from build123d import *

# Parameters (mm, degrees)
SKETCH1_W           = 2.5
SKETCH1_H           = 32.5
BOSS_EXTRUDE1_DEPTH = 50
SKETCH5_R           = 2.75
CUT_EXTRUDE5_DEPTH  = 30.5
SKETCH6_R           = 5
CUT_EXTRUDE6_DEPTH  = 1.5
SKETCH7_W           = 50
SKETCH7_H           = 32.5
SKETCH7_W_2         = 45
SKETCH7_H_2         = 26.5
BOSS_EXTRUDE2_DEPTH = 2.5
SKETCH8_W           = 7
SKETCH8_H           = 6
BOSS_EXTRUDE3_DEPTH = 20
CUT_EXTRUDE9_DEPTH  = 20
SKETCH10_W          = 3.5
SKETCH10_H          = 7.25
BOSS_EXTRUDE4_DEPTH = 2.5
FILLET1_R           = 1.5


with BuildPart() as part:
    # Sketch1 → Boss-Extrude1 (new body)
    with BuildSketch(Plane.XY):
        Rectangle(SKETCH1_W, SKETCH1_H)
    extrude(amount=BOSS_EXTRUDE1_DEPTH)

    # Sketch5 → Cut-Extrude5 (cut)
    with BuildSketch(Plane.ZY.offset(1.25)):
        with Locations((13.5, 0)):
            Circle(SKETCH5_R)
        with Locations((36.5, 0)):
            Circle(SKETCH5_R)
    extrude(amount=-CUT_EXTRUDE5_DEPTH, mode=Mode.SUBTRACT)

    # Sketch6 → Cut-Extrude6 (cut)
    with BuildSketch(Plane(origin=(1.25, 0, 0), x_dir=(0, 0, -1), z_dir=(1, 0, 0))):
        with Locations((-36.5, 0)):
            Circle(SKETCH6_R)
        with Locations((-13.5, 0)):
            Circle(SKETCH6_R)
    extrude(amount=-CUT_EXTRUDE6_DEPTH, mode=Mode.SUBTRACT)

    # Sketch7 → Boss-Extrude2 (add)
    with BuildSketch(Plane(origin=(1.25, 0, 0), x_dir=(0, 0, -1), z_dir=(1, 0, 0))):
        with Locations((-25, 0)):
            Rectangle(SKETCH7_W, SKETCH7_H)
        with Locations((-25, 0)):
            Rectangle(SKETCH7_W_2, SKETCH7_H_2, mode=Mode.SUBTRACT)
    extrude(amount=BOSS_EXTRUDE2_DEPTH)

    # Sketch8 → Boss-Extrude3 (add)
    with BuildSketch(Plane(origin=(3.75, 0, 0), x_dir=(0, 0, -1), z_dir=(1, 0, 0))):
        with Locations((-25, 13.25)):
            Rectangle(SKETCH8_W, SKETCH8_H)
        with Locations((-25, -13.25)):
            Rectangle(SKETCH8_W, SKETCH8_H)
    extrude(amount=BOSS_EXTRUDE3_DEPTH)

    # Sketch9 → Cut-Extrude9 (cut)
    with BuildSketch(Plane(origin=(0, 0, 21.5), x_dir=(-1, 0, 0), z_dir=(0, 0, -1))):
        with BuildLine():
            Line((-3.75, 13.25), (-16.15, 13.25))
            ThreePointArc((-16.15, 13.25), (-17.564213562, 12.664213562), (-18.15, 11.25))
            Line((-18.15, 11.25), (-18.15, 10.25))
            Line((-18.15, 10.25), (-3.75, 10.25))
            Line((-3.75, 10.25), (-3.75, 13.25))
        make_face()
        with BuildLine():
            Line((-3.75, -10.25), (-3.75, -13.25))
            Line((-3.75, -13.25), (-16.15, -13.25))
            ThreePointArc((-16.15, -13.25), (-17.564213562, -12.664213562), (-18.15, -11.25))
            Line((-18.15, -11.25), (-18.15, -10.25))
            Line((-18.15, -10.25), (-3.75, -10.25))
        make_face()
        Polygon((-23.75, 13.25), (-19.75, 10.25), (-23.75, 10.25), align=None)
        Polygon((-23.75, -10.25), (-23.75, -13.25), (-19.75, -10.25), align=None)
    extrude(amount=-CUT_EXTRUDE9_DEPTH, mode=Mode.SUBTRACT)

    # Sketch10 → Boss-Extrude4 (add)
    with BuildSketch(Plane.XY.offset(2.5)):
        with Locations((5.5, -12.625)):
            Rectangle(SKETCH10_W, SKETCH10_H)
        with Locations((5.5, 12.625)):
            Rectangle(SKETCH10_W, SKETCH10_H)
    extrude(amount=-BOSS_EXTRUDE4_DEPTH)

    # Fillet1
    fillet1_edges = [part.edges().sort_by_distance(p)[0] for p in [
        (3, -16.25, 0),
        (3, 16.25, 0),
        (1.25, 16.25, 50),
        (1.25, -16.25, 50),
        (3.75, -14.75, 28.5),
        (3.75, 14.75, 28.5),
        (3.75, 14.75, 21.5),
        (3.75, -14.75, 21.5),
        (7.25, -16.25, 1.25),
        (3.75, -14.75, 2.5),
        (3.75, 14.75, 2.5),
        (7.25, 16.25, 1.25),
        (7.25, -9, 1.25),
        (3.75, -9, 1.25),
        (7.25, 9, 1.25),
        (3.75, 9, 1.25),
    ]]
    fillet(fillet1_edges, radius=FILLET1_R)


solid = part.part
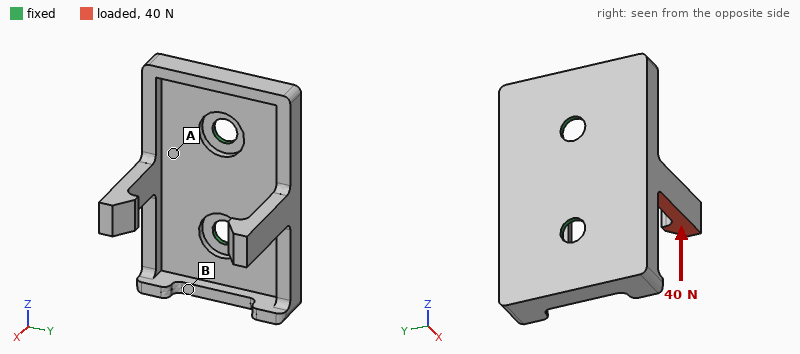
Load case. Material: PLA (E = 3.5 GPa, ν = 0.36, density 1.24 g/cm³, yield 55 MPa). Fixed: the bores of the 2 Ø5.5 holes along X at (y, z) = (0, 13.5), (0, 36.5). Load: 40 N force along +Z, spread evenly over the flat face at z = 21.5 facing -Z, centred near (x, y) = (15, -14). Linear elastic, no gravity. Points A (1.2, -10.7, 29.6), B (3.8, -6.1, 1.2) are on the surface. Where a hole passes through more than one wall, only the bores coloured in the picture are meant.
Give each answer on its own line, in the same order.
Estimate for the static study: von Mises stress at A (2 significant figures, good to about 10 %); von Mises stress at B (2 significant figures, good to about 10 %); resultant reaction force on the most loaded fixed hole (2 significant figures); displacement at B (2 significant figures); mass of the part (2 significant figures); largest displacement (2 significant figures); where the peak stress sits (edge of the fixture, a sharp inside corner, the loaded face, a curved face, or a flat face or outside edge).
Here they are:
8.2 MPa
3.0 MPa
41 N
0.13 mm
7.4 g
0.66 mm
a curved face
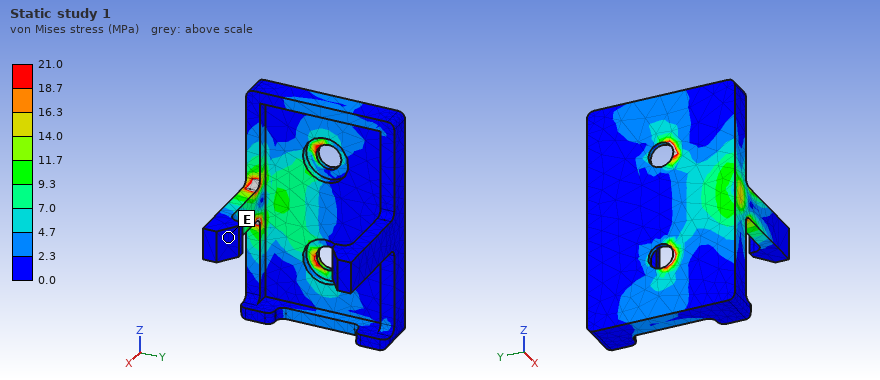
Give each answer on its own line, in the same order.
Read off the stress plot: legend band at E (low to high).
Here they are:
0.0 to 2.3 MPa
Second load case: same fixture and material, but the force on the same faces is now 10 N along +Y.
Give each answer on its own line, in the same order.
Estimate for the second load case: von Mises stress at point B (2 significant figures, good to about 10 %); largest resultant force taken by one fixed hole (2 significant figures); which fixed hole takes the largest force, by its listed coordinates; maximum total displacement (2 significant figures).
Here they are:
2.2 MPa
7.4 N
(0, 13.5)
0.76 mm
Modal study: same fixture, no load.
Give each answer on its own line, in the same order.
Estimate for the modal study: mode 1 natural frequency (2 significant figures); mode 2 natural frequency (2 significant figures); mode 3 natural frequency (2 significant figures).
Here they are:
680 Hz
980 Hz
1300 Hz
